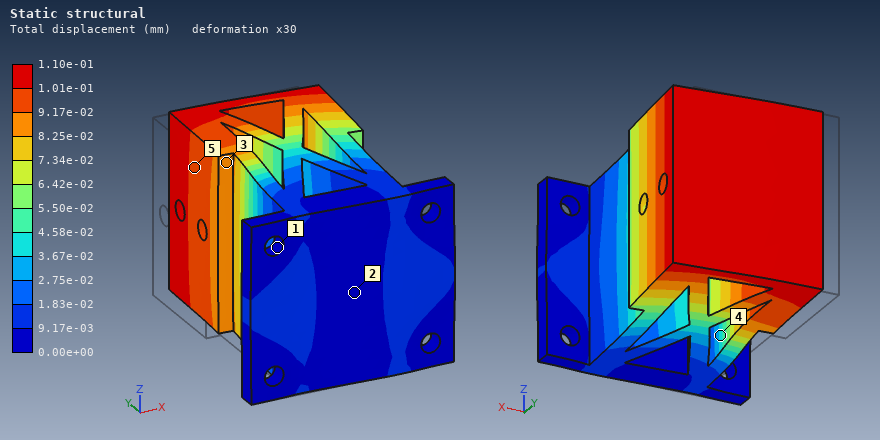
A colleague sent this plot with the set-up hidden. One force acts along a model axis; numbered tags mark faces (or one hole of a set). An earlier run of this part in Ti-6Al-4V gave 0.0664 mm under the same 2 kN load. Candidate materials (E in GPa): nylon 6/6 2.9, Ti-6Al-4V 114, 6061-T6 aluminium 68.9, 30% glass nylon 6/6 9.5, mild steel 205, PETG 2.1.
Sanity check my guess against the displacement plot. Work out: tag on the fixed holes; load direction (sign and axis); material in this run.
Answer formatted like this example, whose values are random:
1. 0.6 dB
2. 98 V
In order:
1. 1
2. +X
3. 6061-T6 aluminium
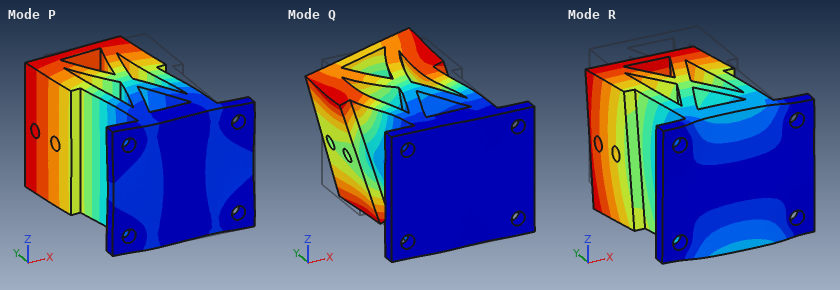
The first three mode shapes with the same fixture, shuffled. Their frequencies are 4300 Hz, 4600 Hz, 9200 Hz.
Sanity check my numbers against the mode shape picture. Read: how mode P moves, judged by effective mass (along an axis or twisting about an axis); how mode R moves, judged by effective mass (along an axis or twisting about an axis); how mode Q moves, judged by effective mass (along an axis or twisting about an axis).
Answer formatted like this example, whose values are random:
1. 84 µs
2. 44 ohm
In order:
1. along X
2. along Z
3. twisting about Y
